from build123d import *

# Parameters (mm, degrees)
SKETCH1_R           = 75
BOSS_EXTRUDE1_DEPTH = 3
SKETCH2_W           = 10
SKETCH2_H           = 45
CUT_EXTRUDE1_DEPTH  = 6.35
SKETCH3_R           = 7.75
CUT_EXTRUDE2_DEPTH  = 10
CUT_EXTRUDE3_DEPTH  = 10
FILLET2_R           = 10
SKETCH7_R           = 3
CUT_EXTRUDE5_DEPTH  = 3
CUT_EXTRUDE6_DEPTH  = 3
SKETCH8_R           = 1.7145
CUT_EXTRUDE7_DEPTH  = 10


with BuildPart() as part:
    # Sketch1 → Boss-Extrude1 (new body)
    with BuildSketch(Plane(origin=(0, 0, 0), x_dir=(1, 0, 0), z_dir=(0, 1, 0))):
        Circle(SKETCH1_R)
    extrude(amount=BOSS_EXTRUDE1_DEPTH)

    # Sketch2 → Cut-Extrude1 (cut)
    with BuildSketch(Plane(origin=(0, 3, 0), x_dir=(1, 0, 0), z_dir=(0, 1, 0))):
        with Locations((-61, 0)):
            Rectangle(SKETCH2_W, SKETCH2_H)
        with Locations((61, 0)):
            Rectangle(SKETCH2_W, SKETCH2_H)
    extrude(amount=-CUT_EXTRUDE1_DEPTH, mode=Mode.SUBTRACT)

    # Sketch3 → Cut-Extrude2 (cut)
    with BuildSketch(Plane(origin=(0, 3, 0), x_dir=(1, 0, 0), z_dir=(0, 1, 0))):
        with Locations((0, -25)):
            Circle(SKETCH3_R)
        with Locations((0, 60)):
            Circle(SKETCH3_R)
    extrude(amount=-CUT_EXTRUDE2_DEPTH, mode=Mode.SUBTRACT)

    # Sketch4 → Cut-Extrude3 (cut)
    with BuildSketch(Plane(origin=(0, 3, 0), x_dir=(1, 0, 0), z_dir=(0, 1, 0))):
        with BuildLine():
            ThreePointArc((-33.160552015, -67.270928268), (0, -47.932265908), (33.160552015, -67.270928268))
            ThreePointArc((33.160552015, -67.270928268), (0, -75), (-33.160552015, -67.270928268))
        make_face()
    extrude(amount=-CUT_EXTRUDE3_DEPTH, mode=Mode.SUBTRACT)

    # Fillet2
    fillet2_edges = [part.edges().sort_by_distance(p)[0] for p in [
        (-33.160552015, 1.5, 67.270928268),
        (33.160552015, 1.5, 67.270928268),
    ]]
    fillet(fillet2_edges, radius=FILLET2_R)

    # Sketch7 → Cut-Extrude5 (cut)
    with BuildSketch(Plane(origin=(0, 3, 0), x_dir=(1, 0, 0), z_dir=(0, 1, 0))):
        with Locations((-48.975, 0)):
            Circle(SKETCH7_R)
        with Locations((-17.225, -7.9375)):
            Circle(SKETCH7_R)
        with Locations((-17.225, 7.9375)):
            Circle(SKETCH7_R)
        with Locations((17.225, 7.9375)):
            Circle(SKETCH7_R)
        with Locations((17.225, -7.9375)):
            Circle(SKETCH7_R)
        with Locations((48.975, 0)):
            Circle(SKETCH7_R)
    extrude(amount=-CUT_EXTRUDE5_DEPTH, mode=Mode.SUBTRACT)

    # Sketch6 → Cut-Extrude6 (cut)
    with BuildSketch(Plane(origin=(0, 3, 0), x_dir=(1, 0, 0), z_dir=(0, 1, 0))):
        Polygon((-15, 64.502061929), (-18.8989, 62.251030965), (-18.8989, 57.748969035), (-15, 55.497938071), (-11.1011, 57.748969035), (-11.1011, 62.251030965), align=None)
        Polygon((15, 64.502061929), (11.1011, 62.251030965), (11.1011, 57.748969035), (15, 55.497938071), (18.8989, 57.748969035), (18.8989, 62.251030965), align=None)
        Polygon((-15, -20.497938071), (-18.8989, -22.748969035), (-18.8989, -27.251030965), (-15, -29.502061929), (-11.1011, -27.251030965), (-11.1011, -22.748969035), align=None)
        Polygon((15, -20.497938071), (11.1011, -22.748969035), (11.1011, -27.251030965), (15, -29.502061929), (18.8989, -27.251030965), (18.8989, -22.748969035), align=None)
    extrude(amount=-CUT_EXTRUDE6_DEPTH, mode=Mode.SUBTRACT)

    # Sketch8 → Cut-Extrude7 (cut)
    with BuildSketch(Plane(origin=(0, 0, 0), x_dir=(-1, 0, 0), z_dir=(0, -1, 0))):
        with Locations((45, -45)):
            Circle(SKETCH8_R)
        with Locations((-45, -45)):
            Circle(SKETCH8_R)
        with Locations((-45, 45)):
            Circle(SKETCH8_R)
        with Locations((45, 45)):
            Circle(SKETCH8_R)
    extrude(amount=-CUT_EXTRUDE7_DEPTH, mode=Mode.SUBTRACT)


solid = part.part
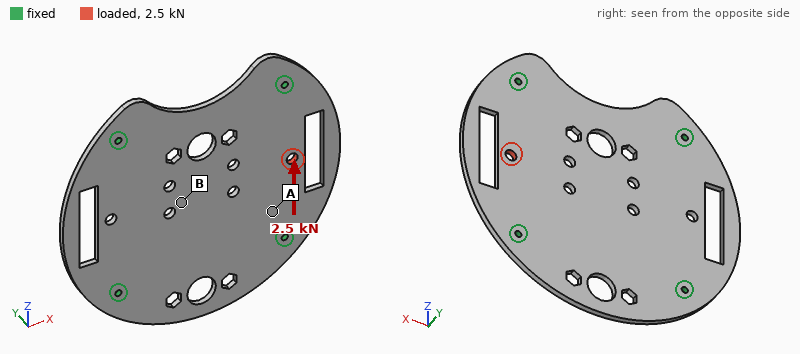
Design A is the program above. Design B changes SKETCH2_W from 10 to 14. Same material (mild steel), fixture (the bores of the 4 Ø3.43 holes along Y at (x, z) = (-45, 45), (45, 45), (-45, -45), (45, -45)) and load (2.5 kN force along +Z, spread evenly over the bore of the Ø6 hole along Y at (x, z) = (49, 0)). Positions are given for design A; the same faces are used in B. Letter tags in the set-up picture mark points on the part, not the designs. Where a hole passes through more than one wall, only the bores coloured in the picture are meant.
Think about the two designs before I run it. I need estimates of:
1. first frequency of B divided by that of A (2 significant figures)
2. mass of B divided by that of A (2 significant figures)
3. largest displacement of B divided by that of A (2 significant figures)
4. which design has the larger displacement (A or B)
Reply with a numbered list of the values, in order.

1. 1.00
2. 0.98
3. 1.2
4. B
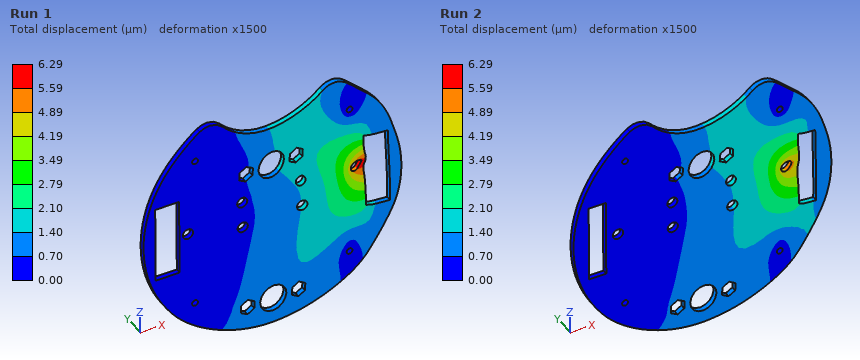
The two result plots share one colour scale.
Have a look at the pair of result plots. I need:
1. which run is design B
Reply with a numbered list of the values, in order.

1. Run 1
